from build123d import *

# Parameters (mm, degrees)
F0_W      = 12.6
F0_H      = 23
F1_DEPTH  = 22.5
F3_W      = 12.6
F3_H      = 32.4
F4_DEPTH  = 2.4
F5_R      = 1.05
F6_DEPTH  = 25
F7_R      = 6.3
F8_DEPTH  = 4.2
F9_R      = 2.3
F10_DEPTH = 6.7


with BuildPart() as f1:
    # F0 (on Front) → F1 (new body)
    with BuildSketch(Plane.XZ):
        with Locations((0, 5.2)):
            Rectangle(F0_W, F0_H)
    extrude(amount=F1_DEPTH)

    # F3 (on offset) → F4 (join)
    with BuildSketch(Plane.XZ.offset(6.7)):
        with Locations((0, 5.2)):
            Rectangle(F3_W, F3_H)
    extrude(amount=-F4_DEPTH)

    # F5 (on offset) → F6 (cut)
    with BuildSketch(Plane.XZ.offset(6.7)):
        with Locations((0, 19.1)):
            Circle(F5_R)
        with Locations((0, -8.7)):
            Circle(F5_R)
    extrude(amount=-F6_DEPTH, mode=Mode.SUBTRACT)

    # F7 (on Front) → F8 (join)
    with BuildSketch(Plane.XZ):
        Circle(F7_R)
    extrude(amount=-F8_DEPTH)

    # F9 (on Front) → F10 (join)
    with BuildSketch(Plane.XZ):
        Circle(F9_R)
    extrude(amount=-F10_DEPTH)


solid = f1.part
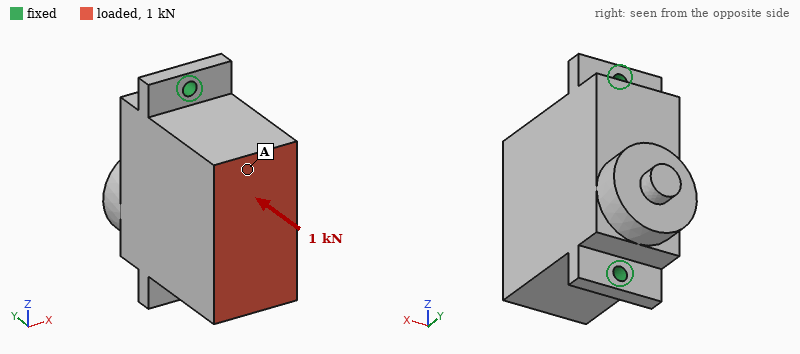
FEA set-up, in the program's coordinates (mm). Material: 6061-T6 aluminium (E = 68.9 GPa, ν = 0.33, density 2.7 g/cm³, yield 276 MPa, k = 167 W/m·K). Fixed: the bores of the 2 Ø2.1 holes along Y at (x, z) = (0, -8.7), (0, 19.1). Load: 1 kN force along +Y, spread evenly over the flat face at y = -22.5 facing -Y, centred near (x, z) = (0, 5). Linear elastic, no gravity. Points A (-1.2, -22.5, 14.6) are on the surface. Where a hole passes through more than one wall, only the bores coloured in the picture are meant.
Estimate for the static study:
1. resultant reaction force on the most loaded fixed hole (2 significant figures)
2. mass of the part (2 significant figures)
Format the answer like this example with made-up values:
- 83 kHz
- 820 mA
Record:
- 500 N
- 20 g
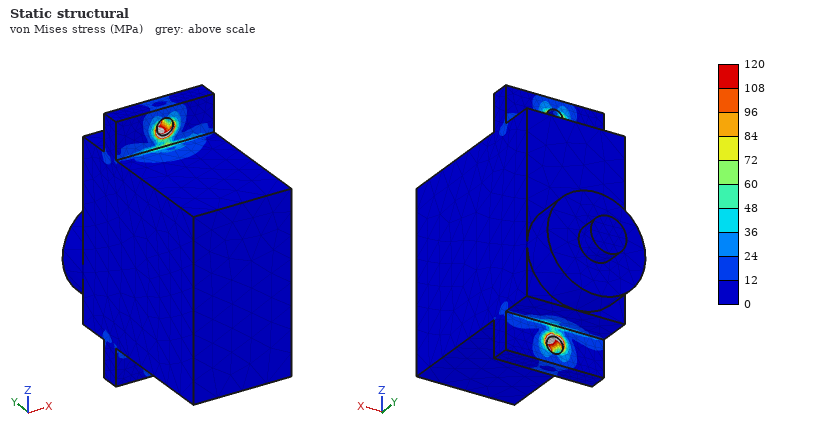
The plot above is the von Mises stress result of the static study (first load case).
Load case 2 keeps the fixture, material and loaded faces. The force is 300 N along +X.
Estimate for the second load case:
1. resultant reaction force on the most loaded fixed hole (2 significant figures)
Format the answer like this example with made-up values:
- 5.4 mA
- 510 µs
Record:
- 150 N
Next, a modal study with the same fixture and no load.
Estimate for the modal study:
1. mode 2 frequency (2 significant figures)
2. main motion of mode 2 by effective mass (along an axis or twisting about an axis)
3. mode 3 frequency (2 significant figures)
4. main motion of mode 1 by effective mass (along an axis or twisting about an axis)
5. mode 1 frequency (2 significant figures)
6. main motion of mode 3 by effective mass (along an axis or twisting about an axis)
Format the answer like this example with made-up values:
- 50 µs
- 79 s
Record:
- 15 kHz
- along Y
- 16 kHz
- along X
- 3700 Hz
- along Z
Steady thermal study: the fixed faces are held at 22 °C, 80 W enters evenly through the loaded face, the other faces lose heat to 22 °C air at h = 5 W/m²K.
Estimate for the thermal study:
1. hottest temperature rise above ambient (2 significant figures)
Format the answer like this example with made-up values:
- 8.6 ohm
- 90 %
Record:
- 68 K
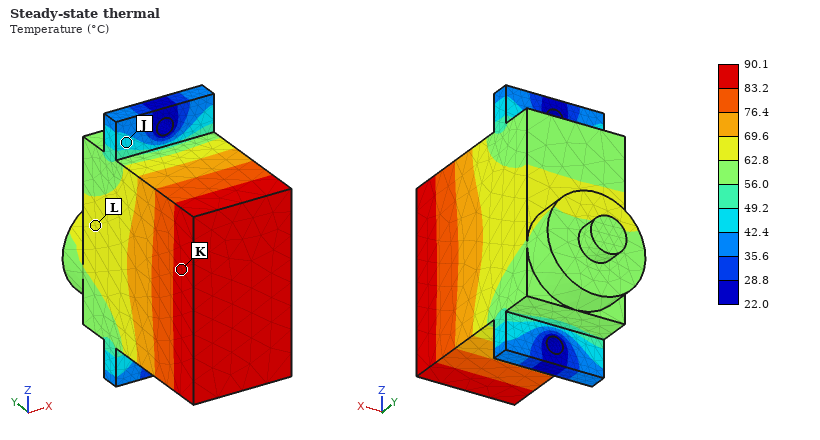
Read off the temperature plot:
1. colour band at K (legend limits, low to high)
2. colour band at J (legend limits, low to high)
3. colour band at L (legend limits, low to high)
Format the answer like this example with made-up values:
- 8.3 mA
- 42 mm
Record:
- 83.2 to 90.1 °C
- 42.4 to 49.2 °C
- 62.8 to 69.6 °C
